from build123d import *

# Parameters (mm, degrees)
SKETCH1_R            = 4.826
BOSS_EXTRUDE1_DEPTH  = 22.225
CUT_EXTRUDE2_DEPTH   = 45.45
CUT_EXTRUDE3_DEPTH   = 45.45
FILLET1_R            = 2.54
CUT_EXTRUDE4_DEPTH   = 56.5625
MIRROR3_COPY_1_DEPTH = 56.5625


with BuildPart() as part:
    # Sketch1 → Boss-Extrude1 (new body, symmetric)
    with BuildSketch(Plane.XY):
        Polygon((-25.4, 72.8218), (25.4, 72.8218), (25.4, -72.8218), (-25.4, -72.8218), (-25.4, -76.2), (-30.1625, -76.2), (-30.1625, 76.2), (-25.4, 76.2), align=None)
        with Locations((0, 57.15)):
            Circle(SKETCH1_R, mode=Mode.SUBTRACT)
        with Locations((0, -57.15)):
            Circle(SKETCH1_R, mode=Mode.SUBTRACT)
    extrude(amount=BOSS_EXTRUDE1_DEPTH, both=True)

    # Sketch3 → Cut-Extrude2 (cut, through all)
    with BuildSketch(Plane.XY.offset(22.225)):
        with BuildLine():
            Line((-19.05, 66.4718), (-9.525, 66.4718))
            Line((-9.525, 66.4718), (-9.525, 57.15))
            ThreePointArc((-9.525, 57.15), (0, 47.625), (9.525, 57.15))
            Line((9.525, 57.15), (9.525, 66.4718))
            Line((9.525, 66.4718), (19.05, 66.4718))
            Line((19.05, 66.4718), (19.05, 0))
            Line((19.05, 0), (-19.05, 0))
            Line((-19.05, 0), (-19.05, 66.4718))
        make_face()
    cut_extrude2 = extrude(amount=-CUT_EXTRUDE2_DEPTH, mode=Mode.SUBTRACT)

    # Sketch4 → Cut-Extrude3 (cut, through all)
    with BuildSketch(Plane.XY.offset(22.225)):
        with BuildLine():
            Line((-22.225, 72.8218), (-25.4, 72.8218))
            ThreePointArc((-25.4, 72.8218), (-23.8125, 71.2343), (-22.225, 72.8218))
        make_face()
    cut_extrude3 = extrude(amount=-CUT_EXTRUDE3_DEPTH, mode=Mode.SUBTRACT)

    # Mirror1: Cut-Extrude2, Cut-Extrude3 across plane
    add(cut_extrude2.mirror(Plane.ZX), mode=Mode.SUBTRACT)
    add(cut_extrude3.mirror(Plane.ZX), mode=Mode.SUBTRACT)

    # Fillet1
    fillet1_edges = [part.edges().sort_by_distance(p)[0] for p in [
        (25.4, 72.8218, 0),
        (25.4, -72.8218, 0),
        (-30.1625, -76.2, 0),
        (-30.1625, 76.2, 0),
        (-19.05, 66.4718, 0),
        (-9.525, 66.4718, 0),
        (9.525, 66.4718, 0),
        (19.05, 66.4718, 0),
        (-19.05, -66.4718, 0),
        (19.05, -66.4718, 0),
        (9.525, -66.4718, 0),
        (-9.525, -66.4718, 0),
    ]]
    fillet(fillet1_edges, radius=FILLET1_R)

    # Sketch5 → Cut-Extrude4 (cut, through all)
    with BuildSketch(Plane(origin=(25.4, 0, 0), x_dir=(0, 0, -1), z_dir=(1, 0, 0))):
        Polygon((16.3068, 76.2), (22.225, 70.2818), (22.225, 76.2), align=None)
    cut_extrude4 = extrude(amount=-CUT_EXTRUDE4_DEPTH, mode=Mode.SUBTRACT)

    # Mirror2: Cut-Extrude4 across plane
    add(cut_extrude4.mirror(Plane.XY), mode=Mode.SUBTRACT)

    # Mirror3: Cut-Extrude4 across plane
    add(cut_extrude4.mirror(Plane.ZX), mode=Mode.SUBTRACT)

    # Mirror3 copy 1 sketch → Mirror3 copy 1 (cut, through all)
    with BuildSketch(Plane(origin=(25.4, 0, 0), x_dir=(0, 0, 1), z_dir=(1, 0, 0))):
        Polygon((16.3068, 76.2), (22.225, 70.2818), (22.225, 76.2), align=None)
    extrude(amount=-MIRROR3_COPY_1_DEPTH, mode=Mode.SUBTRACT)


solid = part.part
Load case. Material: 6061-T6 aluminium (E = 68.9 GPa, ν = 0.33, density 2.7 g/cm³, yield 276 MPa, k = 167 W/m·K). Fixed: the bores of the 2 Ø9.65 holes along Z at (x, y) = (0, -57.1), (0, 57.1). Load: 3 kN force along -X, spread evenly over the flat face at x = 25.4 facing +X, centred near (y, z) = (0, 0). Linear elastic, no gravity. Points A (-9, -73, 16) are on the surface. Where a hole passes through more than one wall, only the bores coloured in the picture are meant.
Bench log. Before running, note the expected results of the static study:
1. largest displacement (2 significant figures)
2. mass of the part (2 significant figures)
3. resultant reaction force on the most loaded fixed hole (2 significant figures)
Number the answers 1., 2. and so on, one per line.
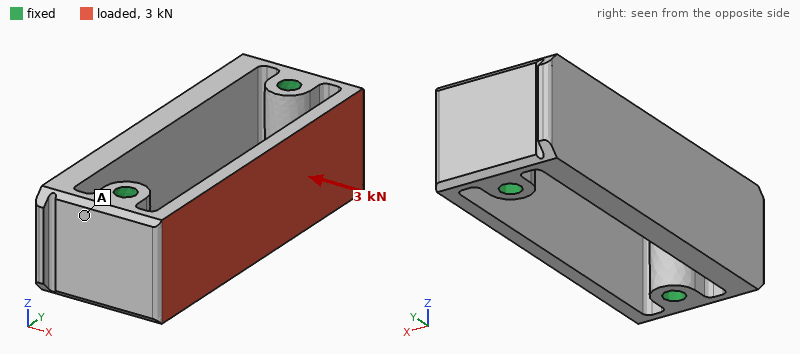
1. 0.37 mm
2. 420 g
3. 2.9 kN
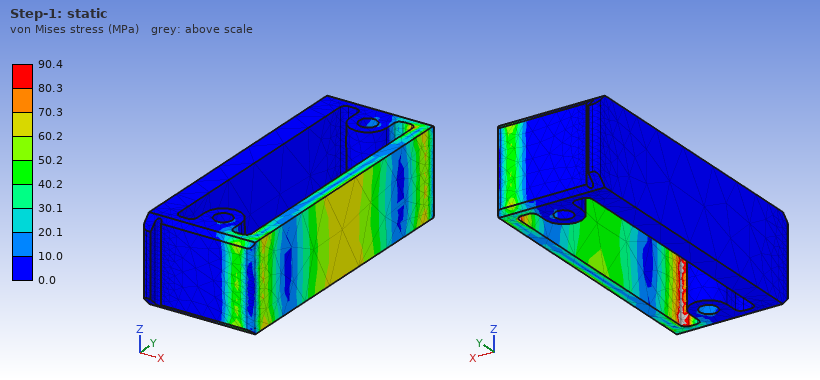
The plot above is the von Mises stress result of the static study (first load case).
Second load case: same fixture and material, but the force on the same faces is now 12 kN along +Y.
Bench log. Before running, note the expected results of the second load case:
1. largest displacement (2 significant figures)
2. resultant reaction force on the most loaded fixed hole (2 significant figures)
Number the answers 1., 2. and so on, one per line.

1. 0.14 mm
2. 6.1 kN
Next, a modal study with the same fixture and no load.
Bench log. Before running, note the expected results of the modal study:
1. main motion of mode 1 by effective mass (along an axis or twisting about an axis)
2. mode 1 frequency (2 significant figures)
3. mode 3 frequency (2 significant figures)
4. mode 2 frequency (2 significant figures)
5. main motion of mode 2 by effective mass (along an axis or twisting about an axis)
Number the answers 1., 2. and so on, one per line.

1. along X
2. 1600 Hz
3. 3500 Hz
4. 2200 Hz
5. along X
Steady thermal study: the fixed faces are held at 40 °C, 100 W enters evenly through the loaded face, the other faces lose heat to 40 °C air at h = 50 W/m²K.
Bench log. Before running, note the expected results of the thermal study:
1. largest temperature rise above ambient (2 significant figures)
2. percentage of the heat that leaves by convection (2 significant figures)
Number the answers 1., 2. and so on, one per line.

1. 45 K
2. 16 %
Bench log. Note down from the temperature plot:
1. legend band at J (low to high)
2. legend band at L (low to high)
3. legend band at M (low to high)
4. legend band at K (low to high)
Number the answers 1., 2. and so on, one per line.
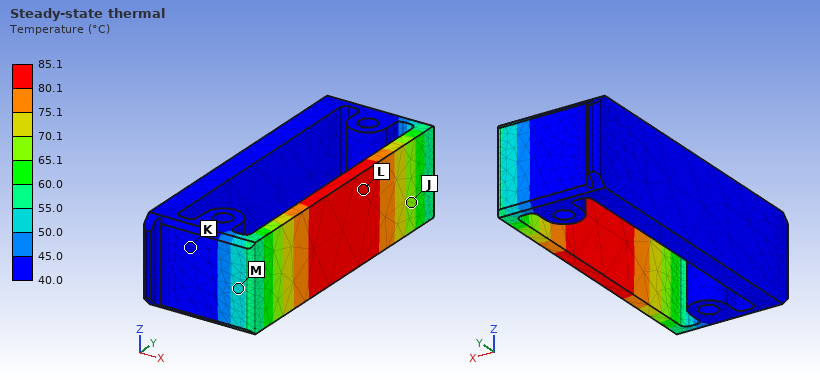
1. 65.1 to 70.1 °C
2. 80.1 to 85.1 °C
3. 50.0 to 55.0 °C
4. 40.0 to 45.0 °C
